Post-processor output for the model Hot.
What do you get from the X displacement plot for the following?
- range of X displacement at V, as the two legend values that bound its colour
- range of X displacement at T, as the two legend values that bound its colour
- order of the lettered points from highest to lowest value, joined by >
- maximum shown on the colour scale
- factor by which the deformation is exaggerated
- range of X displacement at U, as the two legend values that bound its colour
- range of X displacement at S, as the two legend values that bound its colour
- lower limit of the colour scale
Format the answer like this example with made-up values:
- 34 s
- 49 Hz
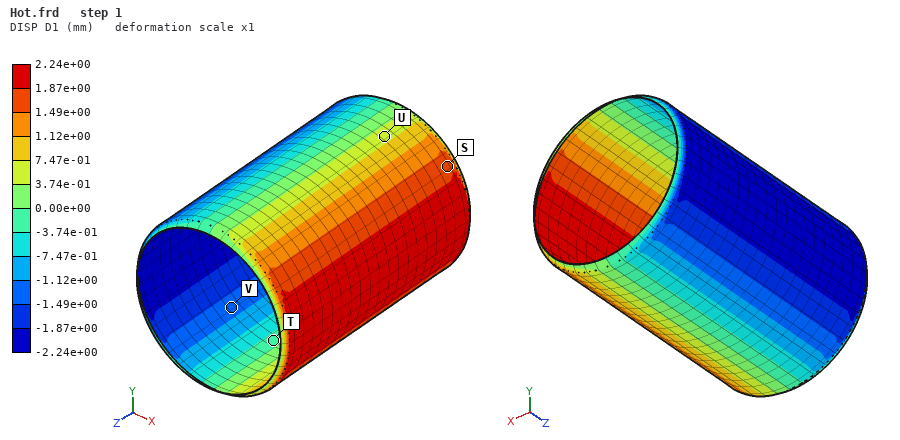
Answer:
- -1.49e+00 to -1.12e+00 mm
- -3.74e-01 to 0.00e+00 mm
- S > U > T > V
- 2.24e+00 mm
- 1
- 3.74e-01 to 7.47e-01 mm
- 1.49e+00 to 1.87e+00 mm
- -2.24e+00 mm
